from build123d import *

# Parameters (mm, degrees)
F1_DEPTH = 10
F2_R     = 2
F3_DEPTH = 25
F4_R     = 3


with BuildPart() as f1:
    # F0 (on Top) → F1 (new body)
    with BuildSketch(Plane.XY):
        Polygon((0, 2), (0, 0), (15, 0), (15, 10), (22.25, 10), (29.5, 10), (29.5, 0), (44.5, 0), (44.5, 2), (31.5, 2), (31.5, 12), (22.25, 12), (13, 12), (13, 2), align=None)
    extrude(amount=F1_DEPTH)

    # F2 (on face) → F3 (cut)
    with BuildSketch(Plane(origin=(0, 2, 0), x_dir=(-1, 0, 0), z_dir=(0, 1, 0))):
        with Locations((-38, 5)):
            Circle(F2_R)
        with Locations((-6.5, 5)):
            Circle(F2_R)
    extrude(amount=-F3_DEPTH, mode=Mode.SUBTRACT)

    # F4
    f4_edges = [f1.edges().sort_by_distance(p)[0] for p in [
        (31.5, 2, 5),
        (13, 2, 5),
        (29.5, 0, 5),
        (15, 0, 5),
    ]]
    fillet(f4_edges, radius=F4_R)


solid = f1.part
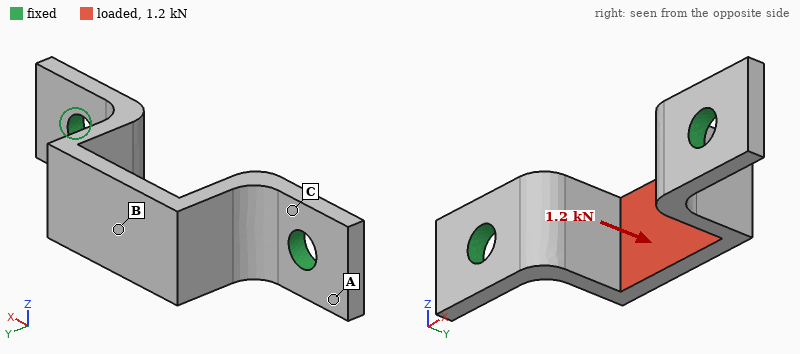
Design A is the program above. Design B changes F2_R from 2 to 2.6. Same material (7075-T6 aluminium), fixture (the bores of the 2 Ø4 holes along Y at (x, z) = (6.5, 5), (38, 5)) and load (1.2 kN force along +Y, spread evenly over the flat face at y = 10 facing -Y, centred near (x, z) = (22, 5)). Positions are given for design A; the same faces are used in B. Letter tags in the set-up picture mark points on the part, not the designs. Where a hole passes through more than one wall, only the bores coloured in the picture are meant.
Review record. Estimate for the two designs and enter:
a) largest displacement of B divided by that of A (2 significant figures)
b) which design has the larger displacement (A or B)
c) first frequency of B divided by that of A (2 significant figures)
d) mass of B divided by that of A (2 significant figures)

0.92
A
1.1
0.97
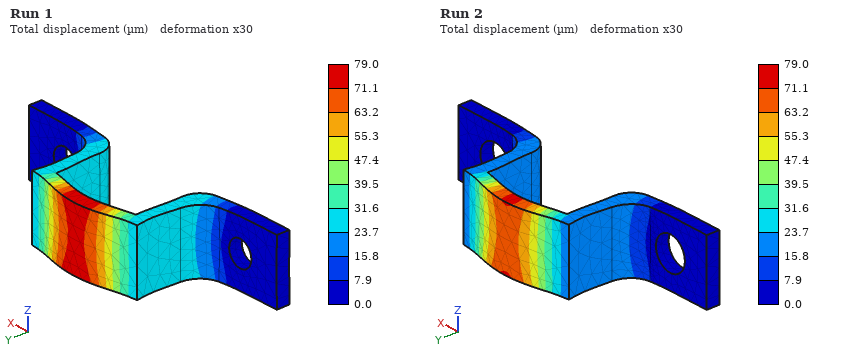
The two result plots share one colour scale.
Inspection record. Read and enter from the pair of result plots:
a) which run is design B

Run 2
